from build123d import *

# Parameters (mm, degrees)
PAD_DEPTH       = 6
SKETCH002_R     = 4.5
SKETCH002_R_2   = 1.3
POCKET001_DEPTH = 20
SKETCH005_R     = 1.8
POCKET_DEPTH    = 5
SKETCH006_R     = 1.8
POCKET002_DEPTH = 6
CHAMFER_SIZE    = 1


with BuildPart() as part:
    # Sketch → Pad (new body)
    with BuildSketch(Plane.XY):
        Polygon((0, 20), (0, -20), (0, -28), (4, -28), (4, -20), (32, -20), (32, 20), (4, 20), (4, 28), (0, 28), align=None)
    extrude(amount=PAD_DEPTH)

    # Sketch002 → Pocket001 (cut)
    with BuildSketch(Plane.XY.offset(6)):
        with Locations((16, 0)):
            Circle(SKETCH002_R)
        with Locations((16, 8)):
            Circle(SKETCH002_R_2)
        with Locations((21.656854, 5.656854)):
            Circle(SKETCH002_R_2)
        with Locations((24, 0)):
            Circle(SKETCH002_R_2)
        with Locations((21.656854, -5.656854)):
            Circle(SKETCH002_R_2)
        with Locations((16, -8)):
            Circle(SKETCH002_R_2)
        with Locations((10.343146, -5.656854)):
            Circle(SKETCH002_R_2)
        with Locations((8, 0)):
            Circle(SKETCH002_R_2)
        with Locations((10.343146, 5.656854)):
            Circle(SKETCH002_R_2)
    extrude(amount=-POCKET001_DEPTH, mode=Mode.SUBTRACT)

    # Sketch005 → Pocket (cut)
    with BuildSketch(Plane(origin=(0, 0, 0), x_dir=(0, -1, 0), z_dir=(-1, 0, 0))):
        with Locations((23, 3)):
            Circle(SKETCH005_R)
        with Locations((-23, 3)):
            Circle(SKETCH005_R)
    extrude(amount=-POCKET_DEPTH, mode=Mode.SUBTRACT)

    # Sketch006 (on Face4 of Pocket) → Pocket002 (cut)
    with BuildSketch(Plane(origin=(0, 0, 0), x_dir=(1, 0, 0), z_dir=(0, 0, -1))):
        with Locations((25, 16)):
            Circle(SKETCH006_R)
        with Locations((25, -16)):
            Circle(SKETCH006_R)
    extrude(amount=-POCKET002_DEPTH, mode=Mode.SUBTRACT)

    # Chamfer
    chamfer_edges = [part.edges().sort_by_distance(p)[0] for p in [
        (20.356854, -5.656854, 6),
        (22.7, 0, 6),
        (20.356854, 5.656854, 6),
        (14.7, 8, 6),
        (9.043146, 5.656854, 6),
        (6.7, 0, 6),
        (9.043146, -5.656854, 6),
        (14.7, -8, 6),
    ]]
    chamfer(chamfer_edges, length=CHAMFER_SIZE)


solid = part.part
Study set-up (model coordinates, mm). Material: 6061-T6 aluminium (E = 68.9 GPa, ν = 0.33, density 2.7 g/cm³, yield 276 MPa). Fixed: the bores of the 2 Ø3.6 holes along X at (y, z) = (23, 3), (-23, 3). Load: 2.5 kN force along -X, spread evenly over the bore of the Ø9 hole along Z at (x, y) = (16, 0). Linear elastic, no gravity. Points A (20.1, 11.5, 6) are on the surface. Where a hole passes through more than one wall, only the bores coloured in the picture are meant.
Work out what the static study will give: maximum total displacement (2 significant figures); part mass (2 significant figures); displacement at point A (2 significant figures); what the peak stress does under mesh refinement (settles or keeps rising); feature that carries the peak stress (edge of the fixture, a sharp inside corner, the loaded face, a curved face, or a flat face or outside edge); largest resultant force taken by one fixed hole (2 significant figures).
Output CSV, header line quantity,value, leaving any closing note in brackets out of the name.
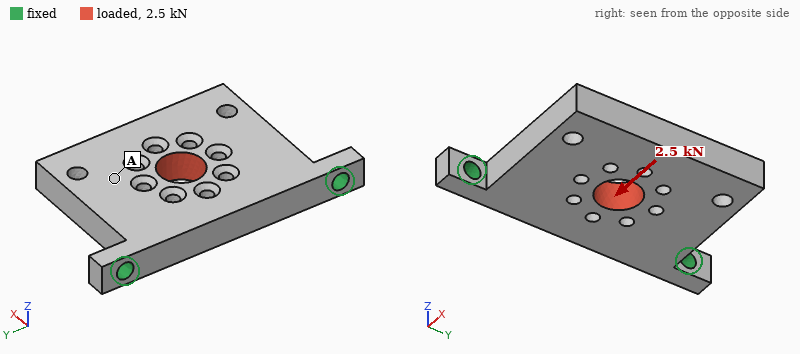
quantity,value
maximum total displacement,22 µm
part mass,19 g
displacement at point A,16 µm
what the peak stress does under mesh refinement,keeps rising
feature that carries the peak stress,edge of the fixture
largest resultant force taken by one fixed hole,1.4 kN
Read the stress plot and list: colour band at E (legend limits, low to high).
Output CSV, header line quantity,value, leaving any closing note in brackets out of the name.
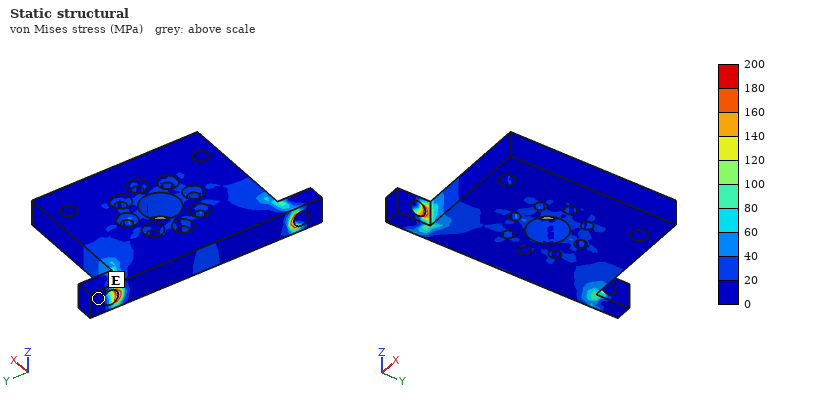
quantity,value
colour band at E,0 to 20 MPa
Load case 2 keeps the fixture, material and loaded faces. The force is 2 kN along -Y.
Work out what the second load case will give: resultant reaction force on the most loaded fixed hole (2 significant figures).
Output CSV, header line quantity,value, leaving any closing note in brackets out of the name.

quantity,value
resultant reaction force on the most loaded fixed hole,1.2 kN
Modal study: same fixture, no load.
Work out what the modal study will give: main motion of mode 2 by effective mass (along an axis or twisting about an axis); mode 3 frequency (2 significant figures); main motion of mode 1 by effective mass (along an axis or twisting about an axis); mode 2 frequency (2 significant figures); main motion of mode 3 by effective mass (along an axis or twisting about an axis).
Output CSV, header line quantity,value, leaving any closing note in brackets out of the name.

quantity,value
main motion of mode 2 by effective mass,twisting about X
mode 3 frequency,12 kHz
main motion of mode 1 by effective mass,along Z
mode 2 frequency,7500 Hz
main motion of mode 3 by effective mass,along Z
